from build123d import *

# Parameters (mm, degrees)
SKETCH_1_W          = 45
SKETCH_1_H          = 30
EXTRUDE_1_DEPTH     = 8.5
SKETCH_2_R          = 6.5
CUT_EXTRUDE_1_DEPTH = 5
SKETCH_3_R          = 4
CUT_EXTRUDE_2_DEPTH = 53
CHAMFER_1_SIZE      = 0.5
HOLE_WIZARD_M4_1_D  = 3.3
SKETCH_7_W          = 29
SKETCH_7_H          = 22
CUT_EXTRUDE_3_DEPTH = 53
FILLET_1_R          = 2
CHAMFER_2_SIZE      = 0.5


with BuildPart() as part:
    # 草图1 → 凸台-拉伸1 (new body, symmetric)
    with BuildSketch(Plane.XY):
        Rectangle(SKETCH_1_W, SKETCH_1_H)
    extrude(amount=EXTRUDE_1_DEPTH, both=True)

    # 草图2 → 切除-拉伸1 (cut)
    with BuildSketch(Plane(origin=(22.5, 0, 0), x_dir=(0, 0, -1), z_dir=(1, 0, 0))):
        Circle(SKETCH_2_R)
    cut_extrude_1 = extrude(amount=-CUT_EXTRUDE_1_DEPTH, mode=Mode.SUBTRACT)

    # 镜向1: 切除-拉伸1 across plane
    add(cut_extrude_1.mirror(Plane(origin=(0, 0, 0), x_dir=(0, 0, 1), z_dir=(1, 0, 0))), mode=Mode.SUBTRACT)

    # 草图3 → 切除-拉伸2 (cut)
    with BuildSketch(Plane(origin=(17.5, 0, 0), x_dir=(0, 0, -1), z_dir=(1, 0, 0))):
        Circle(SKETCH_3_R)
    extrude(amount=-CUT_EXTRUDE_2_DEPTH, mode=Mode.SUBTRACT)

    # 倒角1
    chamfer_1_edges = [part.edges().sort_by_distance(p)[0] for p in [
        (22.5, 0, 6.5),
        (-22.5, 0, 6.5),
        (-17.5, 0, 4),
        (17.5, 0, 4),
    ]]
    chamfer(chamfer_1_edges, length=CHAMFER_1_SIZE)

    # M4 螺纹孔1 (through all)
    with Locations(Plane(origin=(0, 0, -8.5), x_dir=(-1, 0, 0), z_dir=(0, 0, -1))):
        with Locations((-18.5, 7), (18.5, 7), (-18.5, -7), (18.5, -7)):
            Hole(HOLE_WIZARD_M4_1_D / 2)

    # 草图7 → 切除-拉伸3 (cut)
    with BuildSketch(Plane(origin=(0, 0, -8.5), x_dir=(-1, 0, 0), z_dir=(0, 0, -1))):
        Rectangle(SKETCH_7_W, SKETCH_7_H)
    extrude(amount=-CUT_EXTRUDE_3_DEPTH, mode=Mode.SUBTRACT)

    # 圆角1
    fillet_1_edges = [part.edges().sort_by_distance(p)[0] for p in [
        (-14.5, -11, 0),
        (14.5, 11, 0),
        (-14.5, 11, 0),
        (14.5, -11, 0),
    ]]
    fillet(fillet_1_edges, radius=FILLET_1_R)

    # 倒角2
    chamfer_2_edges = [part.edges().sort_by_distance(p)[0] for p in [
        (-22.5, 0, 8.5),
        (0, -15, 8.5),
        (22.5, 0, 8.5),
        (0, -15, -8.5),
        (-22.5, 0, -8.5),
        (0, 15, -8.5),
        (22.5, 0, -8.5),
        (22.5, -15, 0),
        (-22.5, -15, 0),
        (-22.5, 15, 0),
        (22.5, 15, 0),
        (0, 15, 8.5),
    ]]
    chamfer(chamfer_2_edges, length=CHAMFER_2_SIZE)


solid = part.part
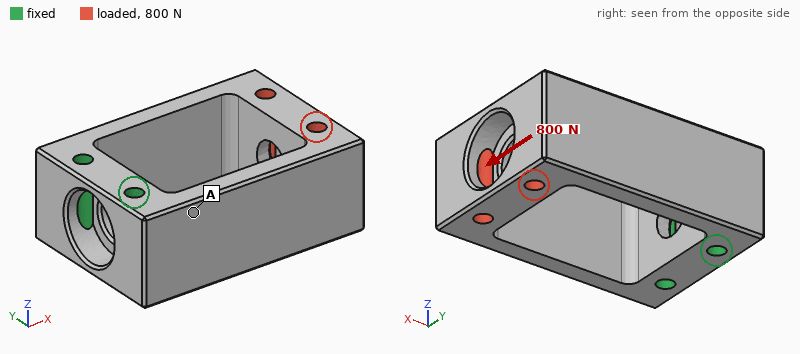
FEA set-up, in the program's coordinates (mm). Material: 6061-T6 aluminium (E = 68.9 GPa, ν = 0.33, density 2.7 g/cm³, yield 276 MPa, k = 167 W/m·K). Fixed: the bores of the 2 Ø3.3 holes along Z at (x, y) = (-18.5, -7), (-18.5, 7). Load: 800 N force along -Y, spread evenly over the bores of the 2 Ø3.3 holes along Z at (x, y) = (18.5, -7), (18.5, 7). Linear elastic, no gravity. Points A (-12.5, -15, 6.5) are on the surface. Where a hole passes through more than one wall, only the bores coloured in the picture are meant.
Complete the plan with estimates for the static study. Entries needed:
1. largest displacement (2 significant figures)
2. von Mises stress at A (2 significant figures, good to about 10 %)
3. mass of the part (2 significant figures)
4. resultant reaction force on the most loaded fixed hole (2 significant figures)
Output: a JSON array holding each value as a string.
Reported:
["0.23 mm", "110 MPa", "27 g", "910 N"]
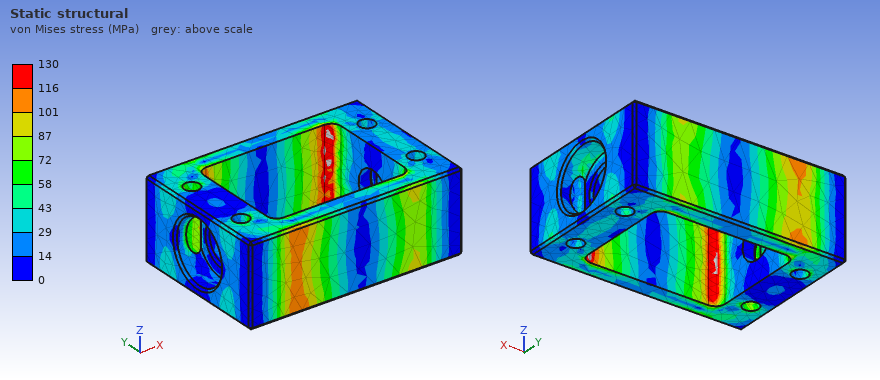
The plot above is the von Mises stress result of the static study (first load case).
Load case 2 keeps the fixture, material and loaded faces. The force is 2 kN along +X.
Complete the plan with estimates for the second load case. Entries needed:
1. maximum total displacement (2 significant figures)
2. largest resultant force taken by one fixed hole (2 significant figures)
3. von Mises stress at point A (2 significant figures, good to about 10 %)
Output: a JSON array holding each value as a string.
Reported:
["33 µm", "1.0 kN", "18 MPa"]
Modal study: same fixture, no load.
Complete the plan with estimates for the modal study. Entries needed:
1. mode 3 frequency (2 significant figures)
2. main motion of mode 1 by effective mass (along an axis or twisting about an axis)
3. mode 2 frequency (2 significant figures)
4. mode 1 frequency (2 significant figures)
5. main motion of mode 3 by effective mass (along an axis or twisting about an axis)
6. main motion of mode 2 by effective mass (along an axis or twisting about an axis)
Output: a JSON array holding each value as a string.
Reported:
["7000 Hz", "along Y", "4500 Hz", "2800 Hz", "twisting about X", "along Z"]
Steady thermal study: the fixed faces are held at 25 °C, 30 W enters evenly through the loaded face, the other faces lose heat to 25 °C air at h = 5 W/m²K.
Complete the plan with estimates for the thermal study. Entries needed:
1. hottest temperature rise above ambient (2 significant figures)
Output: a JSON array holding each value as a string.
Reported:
["50 K"]
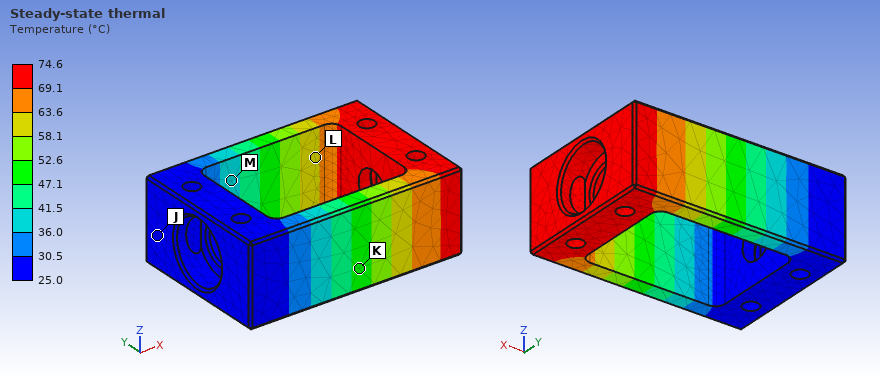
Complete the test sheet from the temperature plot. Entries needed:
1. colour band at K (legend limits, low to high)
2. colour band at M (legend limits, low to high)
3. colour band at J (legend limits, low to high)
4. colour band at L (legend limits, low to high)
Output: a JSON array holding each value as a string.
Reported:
["47.1 to 52.6 °C", "36.0 to 41.5 °C", "25.0 to 30.5 °C", "58.1 to 63.6 °C"]
